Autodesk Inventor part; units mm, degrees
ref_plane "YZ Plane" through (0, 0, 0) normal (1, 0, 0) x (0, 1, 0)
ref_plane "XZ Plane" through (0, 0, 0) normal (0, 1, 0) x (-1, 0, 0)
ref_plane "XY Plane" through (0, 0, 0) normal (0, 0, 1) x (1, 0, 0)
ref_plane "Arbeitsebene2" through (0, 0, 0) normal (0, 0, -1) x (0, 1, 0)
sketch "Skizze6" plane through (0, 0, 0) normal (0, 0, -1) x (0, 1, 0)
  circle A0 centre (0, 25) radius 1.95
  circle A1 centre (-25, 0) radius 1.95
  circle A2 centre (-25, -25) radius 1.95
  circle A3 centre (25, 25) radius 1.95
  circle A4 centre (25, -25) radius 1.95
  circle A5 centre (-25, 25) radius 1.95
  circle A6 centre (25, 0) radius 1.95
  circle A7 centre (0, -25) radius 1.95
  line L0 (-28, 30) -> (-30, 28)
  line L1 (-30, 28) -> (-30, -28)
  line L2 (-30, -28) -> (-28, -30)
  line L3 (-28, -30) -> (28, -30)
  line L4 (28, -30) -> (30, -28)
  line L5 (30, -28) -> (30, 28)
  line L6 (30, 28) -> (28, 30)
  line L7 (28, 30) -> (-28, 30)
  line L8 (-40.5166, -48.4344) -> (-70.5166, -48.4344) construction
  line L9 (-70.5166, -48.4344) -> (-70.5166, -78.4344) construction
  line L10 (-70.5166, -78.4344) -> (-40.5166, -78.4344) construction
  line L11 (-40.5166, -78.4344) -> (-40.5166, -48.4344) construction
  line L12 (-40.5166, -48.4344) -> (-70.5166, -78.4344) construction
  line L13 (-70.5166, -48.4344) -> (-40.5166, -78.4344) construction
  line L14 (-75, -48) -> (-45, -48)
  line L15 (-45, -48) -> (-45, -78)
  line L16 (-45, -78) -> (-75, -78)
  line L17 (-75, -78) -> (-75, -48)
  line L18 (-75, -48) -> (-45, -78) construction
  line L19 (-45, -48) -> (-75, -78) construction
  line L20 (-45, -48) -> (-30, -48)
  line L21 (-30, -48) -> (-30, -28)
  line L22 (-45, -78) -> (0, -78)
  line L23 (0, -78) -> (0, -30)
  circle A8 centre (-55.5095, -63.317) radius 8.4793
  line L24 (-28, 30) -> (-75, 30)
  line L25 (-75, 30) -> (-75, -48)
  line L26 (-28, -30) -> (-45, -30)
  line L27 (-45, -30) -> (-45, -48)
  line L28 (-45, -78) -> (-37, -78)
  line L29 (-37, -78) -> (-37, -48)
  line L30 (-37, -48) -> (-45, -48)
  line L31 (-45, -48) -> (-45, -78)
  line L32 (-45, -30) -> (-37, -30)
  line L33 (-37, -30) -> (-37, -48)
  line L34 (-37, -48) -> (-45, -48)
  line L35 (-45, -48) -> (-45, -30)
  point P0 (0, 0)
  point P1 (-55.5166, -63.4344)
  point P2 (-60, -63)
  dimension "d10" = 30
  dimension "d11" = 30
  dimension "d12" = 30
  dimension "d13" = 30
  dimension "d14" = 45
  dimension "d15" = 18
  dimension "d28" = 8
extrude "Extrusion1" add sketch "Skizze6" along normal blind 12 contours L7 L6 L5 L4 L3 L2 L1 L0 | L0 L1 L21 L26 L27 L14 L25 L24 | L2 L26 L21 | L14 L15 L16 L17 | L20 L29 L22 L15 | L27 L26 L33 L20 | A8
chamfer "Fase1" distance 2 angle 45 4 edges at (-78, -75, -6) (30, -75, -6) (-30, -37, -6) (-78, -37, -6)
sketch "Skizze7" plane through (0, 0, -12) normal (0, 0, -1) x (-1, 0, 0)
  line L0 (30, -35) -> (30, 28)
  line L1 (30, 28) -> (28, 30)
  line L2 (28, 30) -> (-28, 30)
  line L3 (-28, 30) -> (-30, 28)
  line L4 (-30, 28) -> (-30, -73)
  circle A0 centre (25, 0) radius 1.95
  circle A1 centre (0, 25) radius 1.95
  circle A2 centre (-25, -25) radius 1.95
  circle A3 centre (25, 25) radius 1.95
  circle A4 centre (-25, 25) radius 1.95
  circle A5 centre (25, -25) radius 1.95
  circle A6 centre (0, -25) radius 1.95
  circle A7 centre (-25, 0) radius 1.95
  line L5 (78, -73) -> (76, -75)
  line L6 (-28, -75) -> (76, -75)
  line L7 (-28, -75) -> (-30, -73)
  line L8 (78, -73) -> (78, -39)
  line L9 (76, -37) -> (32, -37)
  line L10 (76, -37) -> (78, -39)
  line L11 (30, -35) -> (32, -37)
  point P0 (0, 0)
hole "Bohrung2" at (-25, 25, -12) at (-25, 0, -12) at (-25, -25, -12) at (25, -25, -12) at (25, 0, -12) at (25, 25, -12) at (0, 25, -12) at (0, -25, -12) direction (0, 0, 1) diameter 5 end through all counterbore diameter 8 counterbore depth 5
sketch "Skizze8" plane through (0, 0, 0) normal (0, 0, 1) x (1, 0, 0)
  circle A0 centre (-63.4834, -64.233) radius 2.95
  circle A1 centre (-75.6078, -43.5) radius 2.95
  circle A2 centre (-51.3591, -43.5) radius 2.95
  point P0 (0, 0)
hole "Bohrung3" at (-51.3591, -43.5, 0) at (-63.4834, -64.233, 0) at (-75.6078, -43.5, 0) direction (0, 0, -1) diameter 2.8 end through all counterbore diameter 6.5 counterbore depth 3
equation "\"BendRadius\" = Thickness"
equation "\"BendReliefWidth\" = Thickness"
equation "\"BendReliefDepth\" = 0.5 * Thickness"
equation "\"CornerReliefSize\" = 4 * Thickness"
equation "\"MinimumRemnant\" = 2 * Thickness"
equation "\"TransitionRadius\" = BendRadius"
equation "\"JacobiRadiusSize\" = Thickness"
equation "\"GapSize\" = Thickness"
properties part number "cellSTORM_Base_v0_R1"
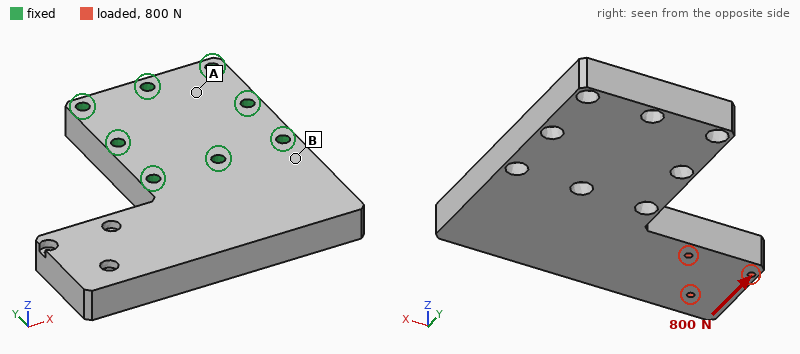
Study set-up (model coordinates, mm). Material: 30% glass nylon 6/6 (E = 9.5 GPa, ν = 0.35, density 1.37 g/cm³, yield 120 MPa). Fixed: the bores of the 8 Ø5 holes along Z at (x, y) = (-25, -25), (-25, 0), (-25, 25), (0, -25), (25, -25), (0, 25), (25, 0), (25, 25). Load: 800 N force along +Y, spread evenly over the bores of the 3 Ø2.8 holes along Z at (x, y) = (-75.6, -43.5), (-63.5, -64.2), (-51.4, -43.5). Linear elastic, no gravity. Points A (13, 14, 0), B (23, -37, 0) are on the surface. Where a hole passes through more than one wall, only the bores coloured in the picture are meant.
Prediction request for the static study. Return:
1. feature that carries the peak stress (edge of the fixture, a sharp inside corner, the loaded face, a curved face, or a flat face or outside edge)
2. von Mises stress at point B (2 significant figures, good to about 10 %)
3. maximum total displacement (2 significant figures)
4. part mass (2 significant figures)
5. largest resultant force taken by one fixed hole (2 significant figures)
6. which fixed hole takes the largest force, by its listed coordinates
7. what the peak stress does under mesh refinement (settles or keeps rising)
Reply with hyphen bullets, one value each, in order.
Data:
- edge of the fixture
- 5.8 MPa
- 0.20 mm
- 130 g
- 1.1 kN
- (-25, -25)
- keeps rising
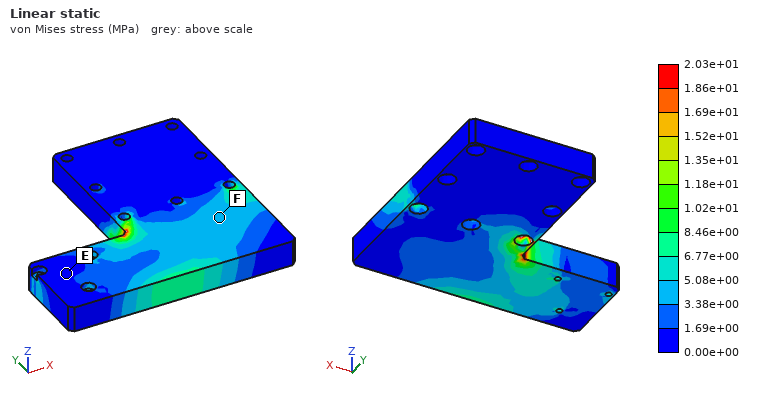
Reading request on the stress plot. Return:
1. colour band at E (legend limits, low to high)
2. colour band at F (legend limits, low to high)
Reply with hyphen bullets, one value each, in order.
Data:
- 0.00e+00 to 1.69e+00 MPa
- 3.38e+00 to 5.08e+00 MPa
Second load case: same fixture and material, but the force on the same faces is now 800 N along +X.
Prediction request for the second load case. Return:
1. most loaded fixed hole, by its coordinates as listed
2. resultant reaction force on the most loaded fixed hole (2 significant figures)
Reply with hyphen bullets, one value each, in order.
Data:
- (-25, -25)
- 460 N
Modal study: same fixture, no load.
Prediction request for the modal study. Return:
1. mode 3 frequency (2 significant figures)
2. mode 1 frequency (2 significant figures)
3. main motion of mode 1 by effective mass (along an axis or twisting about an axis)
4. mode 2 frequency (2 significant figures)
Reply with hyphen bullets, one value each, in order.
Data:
- 2500 Hz
- 870 Hz
- along Z
- 1600 Hz
